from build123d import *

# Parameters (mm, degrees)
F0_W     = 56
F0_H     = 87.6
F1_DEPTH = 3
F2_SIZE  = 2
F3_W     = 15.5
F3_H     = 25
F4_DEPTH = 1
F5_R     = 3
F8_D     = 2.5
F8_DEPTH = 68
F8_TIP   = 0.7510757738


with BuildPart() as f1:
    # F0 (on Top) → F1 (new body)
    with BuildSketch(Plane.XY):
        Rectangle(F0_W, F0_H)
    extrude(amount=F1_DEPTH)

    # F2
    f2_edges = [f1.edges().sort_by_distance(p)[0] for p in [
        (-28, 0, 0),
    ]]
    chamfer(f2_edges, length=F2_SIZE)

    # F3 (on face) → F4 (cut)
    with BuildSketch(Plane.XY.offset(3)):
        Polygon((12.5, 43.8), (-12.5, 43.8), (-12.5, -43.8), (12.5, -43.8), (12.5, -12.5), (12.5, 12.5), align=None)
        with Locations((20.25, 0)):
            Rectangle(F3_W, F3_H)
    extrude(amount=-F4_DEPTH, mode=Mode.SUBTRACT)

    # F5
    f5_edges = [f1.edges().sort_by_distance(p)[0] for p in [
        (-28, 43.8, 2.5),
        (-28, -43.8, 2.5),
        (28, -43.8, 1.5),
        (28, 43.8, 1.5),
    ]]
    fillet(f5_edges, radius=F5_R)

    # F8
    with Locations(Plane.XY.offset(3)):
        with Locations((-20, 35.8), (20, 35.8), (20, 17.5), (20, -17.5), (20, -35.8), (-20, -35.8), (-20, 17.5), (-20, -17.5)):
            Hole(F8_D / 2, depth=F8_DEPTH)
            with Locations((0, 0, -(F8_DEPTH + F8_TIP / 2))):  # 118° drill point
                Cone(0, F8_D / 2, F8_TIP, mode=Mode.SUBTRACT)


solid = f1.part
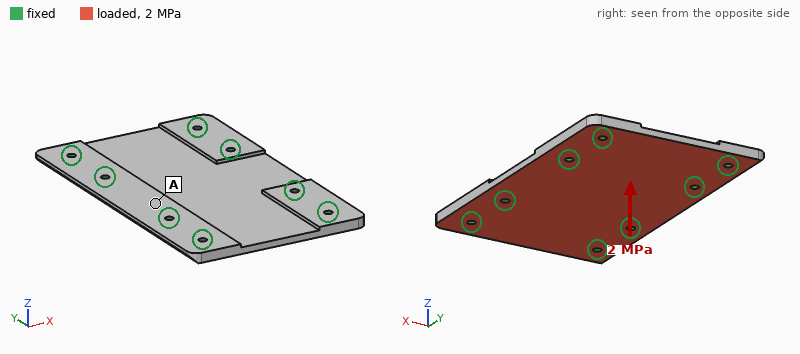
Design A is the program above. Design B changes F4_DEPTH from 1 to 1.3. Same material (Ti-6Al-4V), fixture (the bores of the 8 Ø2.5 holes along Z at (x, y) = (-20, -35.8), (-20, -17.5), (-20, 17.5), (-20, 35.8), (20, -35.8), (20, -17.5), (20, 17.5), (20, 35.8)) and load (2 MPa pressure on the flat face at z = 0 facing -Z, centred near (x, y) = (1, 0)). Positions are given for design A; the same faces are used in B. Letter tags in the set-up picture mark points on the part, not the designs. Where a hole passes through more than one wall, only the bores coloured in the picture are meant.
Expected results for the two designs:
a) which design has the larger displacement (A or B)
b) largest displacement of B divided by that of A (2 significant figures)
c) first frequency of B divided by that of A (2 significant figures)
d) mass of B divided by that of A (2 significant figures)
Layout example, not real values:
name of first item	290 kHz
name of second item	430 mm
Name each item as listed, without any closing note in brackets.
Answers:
which design has the larger displacement	B
largest displacement of B divided by that of A	1.2
first frequency of B divided by that of A	0.98
mass of B divided by that of A	0.93
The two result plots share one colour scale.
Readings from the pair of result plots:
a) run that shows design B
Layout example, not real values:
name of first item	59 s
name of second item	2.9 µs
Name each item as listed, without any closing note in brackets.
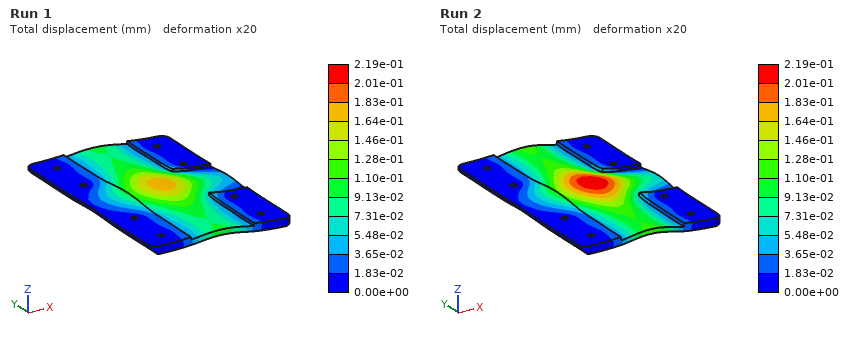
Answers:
run that shows design B	Run 2
